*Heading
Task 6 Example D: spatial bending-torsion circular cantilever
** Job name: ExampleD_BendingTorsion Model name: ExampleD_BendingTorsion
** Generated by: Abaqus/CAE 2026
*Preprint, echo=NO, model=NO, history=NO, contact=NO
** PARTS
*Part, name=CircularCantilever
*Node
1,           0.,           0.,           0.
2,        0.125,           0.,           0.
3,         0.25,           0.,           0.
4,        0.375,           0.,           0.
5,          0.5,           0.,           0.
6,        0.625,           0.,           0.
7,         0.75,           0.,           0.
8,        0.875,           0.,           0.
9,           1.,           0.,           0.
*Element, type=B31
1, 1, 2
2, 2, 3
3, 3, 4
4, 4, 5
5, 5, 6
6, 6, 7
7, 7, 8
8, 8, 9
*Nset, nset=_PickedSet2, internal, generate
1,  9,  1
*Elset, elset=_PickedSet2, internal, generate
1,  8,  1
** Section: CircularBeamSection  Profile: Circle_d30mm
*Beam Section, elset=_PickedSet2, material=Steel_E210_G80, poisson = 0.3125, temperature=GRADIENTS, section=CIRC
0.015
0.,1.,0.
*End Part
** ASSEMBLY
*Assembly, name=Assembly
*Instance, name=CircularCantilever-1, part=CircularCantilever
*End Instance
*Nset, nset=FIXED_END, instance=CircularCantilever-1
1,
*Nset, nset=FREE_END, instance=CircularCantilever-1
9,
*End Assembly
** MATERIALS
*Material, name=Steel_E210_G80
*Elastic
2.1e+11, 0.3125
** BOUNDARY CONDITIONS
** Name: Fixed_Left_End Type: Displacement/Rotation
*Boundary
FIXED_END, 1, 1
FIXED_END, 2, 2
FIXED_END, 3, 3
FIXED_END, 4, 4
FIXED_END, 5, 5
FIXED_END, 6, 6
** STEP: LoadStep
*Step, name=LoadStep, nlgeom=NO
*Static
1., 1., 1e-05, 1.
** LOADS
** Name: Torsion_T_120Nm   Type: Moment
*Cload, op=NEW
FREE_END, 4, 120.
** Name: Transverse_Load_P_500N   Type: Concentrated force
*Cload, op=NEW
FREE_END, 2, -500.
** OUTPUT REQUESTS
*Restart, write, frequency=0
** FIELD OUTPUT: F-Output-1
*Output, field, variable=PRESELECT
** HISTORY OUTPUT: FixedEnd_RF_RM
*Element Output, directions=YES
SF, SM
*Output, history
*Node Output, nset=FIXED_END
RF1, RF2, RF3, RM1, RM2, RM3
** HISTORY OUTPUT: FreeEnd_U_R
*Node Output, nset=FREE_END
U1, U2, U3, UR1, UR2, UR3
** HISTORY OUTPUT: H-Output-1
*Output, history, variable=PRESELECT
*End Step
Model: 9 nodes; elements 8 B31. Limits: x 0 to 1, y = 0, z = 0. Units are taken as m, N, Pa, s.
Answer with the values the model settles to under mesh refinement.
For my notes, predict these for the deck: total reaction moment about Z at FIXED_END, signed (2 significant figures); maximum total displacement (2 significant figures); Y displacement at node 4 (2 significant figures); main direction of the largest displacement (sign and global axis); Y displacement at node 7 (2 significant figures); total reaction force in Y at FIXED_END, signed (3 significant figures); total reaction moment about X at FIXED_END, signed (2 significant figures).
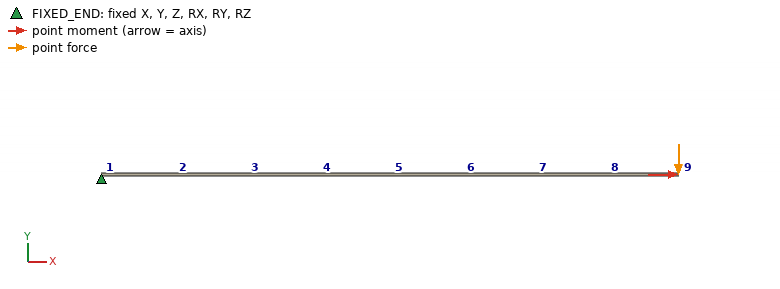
500 N·m
0.020 m
-0.0037 m
-Y
-0.013 m
500 N
-120 N·m
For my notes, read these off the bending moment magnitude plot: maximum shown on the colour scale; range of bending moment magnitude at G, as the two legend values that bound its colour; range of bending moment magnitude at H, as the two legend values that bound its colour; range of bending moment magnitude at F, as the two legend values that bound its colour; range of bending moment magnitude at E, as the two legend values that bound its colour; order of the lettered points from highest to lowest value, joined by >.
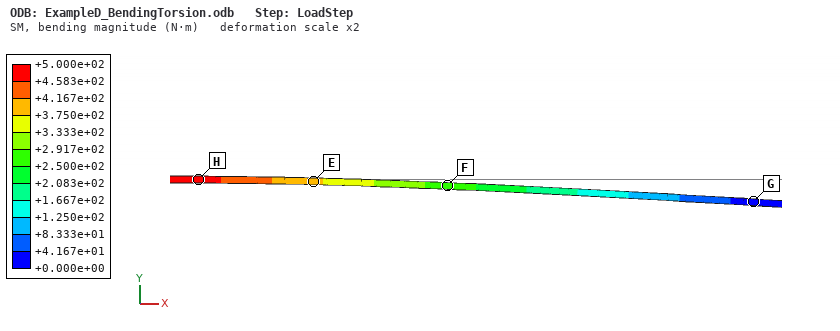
+5.000e+02 N·m
+0.000e+00 to +4.167e+01 N·m
+4.583e+02 to +5.000e+02 N·m
+2.500e+02 to +2.917e+02 N·m
+3.750e+02 to +4.167e+02 N·m
H > E > F > G
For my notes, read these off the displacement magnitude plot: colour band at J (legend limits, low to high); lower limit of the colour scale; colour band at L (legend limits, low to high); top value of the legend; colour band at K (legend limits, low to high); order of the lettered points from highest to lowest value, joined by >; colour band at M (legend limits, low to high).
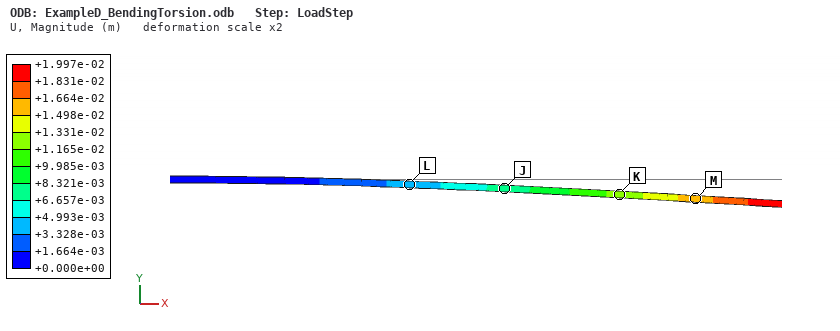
+6.657e-03 to +8.321e-03 m
+0.000e+00 m
+3.328e-03 to +4.993e-03 m
+1.997e-02 m
+1.165e-02 to +1.331e-02 m
M > K > J > L
+1.498e-02 to +1.664e-02 m
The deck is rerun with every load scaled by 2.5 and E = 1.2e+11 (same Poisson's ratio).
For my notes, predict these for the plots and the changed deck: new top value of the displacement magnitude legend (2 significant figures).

0.087 m
